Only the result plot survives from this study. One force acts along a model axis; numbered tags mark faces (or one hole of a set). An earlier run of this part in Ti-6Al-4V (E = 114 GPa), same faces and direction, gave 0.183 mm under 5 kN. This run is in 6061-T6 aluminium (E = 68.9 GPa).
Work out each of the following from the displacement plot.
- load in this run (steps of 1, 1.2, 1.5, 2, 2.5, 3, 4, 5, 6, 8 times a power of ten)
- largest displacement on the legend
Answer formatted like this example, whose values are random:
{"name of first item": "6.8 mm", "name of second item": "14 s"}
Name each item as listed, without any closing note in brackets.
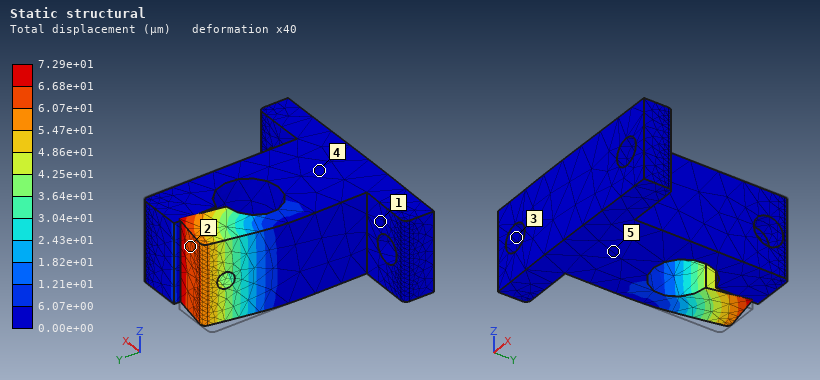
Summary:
{"load in this run": "1.2 kN", "largest displacement on the legend": "7.29e+01 µm"}
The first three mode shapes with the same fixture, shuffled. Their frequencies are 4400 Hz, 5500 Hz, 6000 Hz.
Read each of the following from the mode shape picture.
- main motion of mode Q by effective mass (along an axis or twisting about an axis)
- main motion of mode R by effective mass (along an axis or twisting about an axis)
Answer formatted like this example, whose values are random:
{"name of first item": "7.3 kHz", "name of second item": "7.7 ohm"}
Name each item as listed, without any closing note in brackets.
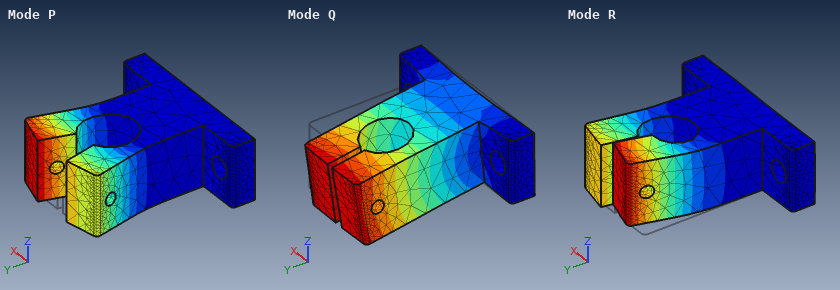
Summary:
{"main motion of mode Q by effective mass": "along Z", "main motion of mode R by effective mass": "along X"}
